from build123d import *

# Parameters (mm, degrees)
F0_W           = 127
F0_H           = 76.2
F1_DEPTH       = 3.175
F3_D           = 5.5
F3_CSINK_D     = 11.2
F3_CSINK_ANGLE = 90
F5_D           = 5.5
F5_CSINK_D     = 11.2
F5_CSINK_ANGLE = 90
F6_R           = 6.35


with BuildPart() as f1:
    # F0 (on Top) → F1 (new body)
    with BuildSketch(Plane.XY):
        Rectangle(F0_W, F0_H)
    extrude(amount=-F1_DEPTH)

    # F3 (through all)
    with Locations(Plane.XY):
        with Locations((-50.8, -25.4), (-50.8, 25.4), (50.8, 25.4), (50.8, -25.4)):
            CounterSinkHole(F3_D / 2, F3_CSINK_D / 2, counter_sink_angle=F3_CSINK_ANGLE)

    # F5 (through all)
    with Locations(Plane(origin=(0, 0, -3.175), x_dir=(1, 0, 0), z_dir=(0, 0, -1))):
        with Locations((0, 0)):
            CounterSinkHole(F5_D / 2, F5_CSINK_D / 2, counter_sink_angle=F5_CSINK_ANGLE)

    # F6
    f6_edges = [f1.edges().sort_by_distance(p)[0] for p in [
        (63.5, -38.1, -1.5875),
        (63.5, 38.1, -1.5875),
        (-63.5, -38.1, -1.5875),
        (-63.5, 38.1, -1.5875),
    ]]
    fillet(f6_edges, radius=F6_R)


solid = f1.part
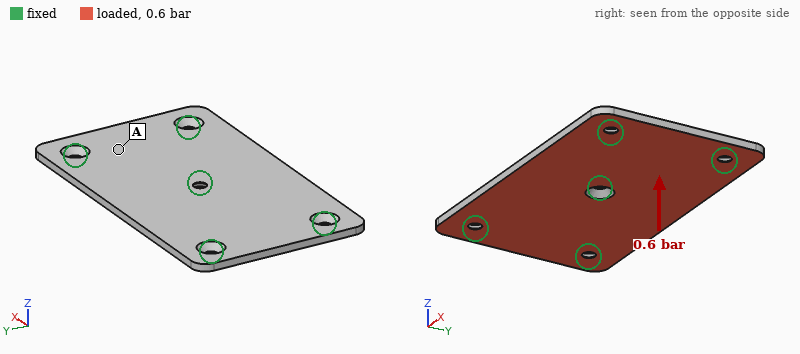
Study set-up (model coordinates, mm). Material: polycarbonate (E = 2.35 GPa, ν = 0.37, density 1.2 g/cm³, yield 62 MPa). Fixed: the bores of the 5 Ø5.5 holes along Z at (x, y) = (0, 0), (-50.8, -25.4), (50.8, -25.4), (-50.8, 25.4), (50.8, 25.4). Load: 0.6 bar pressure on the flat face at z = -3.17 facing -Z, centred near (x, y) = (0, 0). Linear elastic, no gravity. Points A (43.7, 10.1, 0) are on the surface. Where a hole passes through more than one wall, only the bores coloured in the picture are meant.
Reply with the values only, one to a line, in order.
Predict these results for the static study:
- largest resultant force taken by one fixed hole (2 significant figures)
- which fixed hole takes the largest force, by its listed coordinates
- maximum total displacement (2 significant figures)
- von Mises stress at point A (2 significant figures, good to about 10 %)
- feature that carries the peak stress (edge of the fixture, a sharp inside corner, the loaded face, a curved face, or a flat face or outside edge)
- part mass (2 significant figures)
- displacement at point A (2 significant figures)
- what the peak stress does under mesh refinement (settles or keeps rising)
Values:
210 N
(0, 0)
1.5 mm
4.0 MPa
edge of the fixture
36 g
0.26 mm
keeps rising
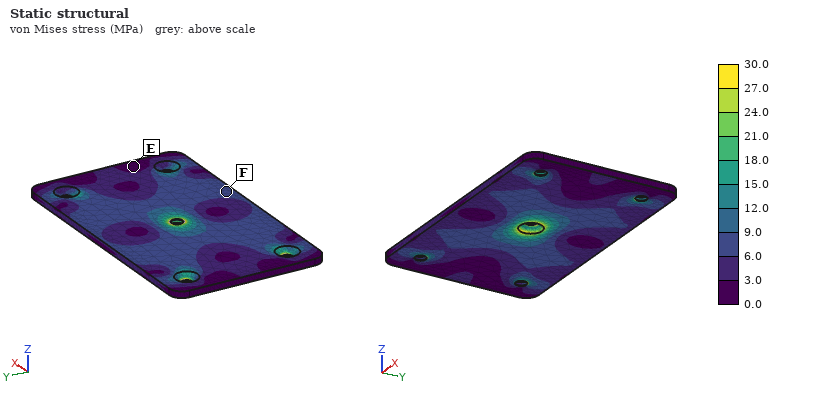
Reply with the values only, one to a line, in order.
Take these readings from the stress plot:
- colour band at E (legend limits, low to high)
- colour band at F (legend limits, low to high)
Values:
0.0 to 3.0 MPa
6.0 to 9.0 MPa
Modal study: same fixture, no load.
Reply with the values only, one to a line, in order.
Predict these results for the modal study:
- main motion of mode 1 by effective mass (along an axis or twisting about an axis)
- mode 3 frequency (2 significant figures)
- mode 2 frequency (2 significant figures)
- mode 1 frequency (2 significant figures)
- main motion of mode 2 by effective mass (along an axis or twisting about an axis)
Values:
twisting about X
920 Hz
670 Hz
550 Hz
along Z
